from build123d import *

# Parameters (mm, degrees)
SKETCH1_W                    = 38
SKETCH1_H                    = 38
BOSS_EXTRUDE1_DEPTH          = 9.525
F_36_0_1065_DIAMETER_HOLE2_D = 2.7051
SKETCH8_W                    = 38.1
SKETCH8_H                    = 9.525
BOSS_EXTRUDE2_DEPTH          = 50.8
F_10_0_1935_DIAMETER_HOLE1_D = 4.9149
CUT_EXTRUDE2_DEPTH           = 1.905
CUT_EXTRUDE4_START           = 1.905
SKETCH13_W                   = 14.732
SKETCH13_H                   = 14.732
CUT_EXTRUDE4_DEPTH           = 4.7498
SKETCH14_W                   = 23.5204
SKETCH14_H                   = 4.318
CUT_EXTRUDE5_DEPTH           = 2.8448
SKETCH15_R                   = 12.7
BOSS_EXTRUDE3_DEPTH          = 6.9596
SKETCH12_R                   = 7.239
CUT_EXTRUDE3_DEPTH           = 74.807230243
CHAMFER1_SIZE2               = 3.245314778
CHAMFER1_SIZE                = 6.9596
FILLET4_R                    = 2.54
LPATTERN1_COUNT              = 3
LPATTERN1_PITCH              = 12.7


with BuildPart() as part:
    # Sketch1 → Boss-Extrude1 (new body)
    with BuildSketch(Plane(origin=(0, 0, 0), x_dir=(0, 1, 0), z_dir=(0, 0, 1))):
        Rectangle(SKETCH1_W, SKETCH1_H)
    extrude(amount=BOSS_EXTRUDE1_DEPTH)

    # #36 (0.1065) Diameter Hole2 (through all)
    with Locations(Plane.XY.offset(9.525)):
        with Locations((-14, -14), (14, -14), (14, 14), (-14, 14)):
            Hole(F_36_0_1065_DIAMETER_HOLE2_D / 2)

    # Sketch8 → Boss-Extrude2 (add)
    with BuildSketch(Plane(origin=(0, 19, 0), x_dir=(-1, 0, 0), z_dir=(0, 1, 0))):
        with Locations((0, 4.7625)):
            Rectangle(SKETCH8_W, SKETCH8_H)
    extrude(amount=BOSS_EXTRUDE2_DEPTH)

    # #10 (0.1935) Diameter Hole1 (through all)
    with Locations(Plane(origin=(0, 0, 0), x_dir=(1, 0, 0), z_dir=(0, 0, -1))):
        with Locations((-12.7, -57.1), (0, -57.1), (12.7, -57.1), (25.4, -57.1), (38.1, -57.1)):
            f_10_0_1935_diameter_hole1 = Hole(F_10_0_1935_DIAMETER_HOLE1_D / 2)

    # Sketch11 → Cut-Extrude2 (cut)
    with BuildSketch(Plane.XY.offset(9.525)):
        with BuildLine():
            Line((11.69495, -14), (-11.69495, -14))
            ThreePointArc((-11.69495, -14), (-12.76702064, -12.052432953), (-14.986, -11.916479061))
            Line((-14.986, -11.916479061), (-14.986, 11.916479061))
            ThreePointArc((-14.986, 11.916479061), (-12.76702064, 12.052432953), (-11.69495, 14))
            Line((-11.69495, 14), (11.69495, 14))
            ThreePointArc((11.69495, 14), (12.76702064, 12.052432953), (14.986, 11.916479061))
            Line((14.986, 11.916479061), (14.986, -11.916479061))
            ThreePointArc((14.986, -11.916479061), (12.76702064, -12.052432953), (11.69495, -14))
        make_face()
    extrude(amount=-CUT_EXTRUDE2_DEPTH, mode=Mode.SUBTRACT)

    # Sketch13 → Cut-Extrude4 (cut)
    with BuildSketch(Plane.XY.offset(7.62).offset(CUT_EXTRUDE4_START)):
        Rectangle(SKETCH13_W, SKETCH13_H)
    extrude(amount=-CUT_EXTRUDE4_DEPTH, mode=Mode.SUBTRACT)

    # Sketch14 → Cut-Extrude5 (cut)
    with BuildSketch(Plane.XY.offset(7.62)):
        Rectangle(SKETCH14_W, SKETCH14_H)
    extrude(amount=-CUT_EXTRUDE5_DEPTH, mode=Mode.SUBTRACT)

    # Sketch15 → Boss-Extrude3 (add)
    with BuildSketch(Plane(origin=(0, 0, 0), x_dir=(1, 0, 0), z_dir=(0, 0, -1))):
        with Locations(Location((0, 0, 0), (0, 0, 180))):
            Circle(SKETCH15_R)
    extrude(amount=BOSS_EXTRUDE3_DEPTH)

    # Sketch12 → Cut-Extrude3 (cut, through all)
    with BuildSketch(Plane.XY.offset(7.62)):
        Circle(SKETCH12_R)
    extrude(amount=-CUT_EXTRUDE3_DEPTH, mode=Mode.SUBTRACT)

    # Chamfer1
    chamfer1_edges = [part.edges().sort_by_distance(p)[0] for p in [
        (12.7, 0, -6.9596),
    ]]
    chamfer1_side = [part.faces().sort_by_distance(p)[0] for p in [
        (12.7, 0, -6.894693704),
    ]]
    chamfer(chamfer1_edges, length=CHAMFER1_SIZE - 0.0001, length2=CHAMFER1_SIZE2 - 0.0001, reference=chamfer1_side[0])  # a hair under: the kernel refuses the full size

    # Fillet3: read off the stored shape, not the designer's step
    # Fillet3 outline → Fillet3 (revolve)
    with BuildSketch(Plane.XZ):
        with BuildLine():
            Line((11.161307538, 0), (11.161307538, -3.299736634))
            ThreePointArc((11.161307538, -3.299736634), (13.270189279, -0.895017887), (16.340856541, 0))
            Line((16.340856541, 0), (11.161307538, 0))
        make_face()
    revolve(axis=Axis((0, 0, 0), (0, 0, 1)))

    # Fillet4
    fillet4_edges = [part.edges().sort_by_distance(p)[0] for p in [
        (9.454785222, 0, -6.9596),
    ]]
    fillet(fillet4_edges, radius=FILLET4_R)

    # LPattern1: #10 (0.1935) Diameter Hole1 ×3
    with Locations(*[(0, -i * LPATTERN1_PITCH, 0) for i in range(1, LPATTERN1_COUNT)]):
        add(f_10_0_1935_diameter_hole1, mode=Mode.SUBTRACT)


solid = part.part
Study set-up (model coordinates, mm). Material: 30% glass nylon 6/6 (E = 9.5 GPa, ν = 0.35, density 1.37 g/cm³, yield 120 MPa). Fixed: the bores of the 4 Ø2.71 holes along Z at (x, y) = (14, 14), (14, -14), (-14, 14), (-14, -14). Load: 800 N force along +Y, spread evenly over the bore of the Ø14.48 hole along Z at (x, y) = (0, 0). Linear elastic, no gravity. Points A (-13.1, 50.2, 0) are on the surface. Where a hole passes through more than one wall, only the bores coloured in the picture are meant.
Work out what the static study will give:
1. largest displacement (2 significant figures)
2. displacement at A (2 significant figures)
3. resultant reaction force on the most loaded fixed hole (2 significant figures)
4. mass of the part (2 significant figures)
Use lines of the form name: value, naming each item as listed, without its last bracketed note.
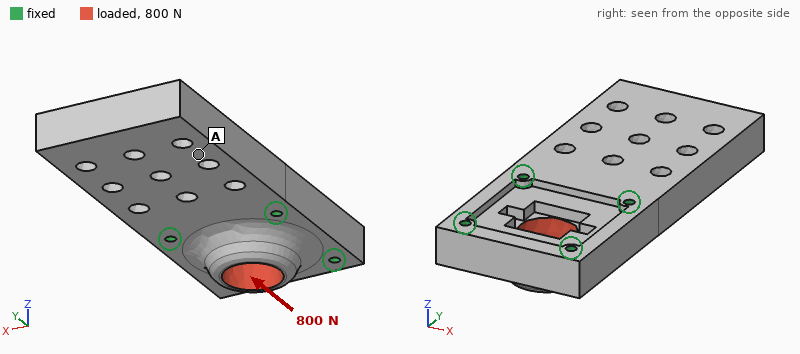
largest displacement: 13 µm
displacement at A: 5.7 µm
resultant reaction force on the most loaded fixed hole: 230 N
mass of the part: 40 g
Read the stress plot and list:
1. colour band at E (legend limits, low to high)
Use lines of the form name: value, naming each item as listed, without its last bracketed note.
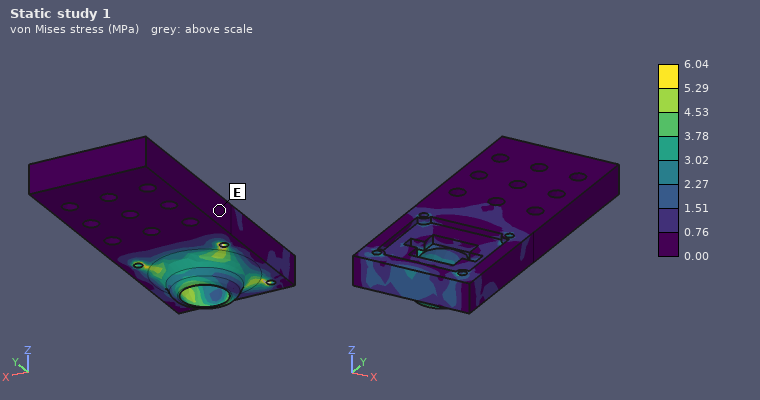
colour band at E: 0.00 to 0.76 MPa
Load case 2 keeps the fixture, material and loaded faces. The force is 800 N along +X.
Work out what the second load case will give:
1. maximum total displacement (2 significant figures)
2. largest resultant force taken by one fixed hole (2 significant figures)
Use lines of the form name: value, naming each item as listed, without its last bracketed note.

maximum total displacement: 12 µm
largest resultant force taken by one fixed hole: 230 N
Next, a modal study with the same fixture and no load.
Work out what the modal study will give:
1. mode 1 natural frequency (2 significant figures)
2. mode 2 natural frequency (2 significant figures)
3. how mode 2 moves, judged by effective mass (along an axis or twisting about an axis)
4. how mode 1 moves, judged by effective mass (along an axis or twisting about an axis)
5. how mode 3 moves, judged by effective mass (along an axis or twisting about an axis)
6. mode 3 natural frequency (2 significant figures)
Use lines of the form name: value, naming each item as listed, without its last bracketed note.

mode 1 natural frequency: 1100 Hz
mode 2 natural frequency: 3400 Hz
how mode 2 moves, judged by effective mass: twisting about Y
how mode 1 moves, judged by effective mass: along Z
how mode 3 moves, judged by effective mass: along X
mode 3 natural frequency: 3700 Hz
